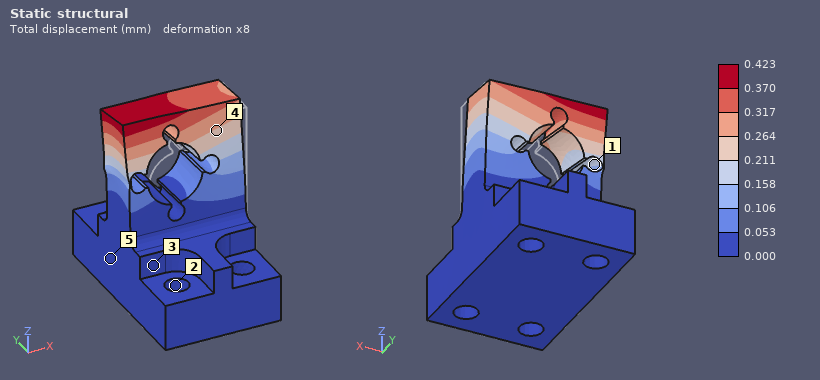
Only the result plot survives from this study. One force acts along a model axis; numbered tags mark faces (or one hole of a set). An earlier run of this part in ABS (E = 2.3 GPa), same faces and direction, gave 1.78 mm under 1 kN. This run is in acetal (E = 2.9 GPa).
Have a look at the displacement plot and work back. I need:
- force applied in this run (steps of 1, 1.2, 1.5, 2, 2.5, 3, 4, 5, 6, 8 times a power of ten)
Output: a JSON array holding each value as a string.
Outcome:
["300 N"]
